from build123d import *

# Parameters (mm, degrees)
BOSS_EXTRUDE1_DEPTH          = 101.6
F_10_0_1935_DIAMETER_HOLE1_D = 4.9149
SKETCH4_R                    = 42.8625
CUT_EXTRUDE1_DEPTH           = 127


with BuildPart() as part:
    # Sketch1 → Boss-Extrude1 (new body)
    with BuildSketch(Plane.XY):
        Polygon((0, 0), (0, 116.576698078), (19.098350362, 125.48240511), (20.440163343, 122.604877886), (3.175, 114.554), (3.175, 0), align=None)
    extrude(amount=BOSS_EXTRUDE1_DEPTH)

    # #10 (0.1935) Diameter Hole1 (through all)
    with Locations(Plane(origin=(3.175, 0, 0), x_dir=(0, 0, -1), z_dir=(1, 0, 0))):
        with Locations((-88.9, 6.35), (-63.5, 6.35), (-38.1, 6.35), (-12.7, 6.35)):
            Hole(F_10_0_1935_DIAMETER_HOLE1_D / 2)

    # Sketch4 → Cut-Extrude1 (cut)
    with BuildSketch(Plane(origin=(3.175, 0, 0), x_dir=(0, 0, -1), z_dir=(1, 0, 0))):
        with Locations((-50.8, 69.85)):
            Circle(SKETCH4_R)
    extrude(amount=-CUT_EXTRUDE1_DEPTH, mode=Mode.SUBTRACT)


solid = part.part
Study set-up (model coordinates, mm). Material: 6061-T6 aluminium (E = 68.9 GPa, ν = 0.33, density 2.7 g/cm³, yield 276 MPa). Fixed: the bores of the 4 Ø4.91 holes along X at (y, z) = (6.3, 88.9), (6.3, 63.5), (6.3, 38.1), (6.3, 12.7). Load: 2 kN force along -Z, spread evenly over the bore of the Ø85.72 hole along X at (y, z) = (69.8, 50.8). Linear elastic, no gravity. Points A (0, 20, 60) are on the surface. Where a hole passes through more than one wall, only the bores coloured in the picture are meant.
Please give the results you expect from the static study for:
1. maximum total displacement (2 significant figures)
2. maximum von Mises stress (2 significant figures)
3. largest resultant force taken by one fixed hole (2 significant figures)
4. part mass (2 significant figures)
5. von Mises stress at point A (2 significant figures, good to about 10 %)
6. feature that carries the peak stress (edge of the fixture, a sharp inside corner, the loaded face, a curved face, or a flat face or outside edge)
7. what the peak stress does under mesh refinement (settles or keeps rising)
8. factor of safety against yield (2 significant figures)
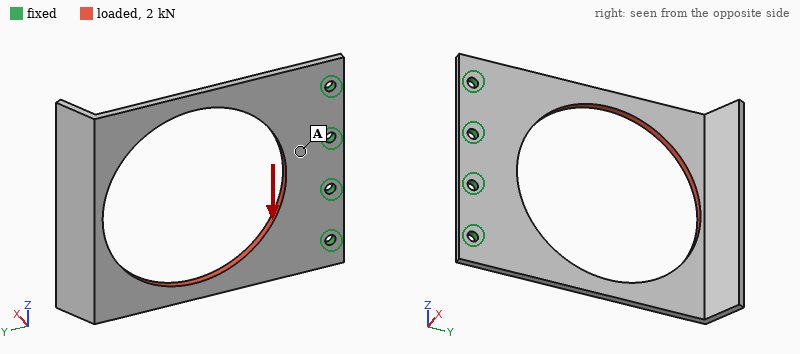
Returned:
0.60 mm
160 MPa
1.8 kN
68 g
26 MPa
the loaded face
settles
1.7
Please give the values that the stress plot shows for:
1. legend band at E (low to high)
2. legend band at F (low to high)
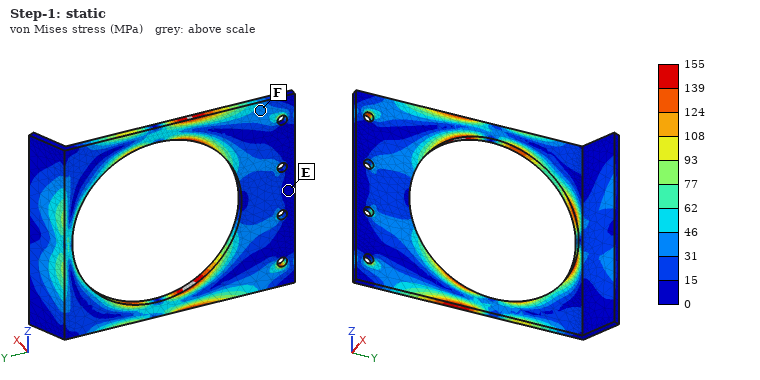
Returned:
0 to 15 MPa
31 to 46 MPa
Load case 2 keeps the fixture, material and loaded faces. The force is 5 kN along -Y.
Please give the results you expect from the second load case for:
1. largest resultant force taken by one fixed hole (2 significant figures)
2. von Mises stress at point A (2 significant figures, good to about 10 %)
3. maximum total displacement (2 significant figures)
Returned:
2.7 kN
16 MPa
0.38 mm
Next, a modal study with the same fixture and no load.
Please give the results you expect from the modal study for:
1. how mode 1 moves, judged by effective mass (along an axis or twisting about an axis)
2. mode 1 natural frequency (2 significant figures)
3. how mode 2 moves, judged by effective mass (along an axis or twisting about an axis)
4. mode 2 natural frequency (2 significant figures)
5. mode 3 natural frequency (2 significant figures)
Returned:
along X
120 Hz
twisting about Y
340 Hz
960 Hz
